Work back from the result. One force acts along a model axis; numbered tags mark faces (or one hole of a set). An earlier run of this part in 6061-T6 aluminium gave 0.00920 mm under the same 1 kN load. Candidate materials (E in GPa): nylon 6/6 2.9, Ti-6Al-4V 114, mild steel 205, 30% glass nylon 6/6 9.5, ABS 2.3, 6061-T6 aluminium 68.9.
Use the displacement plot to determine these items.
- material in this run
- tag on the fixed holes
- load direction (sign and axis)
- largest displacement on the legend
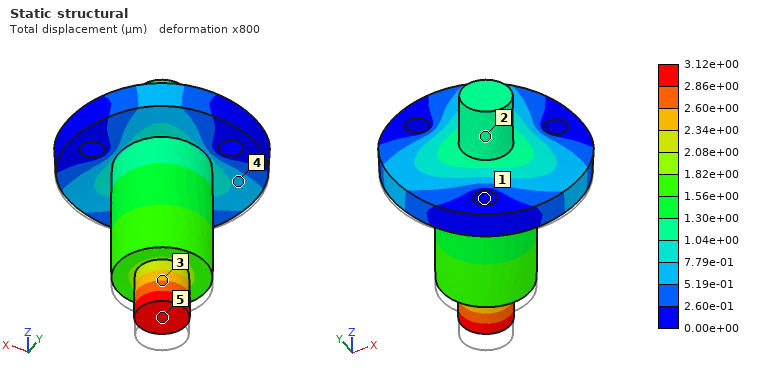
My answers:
mild steel
1
+Z
3.12e+00 µm
